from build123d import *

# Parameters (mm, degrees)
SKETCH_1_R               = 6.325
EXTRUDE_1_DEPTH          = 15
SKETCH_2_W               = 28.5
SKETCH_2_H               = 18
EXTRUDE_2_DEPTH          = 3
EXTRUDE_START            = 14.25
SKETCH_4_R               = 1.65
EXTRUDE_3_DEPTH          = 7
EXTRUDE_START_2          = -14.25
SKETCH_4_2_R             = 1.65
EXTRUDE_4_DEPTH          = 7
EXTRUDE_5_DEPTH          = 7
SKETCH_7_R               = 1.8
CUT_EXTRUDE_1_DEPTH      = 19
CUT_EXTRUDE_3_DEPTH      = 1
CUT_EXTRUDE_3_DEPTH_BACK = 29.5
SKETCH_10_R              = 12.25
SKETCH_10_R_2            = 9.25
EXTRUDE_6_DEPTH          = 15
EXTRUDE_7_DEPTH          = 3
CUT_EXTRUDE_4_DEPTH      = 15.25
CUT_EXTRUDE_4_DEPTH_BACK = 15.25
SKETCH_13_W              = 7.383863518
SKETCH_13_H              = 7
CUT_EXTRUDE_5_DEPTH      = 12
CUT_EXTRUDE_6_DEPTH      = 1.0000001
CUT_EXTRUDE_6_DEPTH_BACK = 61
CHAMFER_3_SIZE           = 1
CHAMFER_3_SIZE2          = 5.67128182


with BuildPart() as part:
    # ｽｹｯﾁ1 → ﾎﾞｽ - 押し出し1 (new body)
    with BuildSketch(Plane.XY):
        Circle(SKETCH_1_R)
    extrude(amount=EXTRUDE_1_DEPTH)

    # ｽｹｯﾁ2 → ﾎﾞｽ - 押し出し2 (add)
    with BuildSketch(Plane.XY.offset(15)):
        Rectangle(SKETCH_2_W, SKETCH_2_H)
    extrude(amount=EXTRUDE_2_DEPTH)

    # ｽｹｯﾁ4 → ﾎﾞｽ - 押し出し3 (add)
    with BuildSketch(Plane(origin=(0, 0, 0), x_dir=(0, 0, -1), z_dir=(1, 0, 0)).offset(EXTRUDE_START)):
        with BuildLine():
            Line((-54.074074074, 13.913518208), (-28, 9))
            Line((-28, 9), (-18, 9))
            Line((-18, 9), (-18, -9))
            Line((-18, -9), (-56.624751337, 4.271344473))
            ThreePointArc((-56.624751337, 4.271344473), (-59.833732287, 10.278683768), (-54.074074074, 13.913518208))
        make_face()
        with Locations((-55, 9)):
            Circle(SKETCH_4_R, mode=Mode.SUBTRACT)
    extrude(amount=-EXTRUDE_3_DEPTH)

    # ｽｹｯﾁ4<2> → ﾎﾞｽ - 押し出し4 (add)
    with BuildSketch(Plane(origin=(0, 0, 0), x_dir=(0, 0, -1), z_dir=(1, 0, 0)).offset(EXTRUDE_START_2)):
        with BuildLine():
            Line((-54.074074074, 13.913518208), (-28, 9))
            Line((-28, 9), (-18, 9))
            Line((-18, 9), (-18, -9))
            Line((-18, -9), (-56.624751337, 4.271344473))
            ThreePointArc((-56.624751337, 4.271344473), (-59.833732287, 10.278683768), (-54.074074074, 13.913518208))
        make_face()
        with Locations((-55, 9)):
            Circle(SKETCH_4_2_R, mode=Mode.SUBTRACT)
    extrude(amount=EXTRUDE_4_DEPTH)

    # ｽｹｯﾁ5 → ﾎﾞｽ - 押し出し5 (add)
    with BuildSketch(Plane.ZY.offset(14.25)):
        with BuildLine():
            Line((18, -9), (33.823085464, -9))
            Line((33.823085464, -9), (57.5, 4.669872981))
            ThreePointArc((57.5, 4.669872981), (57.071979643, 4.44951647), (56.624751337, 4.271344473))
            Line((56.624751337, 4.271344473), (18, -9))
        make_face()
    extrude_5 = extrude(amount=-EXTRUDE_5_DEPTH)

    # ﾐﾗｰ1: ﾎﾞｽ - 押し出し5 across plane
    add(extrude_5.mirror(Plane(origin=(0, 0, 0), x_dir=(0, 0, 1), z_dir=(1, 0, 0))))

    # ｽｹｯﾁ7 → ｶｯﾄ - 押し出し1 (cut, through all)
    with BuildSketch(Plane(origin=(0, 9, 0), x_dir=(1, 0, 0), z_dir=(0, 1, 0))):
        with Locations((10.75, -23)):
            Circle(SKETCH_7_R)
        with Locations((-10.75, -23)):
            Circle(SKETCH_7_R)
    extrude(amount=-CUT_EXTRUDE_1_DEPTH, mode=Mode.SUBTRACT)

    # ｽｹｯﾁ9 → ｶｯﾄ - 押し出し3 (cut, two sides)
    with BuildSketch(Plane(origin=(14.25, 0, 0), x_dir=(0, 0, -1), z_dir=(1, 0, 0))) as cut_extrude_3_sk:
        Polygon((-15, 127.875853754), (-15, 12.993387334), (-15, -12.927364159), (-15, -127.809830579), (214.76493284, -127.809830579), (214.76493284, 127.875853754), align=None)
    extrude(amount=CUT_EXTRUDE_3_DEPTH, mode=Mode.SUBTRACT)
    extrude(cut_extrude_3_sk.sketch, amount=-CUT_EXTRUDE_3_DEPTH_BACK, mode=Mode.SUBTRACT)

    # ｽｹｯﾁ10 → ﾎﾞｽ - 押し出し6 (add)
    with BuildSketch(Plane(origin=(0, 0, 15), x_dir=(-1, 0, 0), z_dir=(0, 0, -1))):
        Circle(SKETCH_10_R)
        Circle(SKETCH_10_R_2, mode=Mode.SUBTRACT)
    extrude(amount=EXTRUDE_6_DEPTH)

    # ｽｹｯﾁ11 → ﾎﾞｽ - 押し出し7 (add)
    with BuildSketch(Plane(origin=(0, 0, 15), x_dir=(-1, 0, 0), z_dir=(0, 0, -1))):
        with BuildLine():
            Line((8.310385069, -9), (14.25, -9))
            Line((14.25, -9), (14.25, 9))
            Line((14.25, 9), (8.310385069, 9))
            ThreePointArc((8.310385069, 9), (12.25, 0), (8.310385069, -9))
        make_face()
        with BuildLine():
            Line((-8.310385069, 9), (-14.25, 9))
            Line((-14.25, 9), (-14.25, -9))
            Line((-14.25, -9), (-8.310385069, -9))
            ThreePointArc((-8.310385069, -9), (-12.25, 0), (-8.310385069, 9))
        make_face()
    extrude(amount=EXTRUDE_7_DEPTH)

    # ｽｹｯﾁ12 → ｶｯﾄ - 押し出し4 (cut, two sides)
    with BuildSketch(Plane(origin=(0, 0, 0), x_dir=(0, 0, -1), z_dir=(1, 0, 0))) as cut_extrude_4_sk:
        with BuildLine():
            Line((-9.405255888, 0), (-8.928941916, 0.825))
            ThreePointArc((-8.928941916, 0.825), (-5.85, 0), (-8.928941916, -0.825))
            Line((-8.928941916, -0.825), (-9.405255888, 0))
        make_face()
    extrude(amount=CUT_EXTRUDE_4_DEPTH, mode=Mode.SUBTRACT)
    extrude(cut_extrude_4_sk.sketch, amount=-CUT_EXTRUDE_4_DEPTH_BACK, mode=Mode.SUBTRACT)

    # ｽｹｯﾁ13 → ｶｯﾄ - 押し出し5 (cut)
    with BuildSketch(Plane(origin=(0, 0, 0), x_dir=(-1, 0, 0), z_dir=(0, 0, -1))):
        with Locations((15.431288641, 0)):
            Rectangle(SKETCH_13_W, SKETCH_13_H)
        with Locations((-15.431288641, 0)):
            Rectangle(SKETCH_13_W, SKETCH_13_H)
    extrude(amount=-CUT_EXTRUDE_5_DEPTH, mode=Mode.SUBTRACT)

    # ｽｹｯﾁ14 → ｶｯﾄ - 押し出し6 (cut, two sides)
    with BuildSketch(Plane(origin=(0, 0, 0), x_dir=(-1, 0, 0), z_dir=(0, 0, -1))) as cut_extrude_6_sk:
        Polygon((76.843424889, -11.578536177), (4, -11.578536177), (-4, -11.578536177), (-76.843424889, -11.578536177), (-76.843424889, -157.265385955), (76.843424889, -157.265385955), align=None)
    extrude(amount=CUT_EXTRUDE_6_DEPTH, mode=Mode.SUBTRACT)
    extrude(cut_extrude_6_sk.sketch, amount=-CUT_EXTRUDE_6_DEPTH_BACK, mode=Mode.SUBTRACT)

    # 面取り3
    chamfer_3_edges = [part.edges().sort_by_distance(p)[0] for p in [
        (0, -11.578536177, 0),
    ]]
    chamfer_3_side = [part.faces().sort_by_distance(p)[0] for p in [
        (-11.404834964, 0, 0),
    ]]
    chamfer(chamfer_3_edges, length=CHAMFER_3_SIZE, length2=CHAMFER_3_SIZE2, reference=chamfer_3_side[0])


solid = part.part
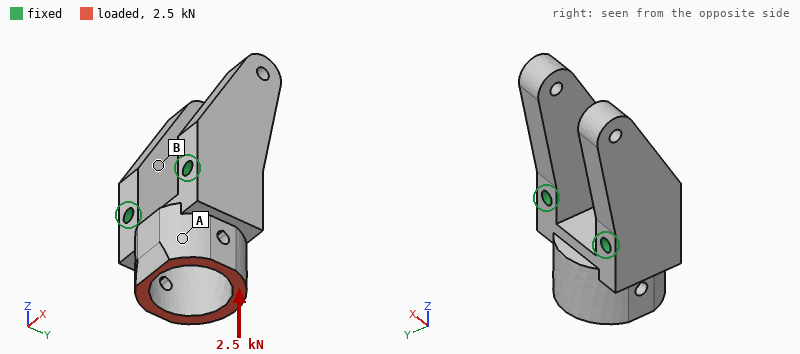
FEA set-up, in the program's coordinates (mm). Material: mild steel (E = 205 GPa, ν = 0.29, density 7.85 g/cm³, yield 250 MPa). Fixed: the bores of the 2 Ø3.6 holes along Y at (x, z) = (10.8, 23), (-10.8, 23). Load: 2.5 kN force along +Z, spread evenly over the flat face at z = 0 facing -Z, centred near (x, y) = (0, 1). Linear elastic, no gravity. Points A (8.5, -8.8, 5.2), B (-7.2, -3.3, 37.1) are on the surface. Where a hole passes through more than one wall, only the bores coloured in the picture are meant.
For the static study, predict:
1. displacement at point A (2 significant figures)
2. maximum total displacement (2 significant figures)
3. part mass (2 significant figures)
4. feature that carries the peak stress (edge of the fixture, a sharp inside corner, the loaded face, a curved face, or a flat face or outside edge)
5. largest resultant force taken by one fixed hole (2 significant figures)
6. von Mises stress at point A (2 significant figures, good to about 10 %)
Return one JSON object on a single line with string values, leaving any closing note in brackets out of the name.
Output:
{"displacement at point A": "1.3 µm", "maximum total displacement": "4.3 µm", "part mass": "100 g", "feature that carries the peak stress": "a curved face", "largest resultant force taken by one fixed hole": "1.3 kN", "von Mises stress at point A": "16 MPa"}
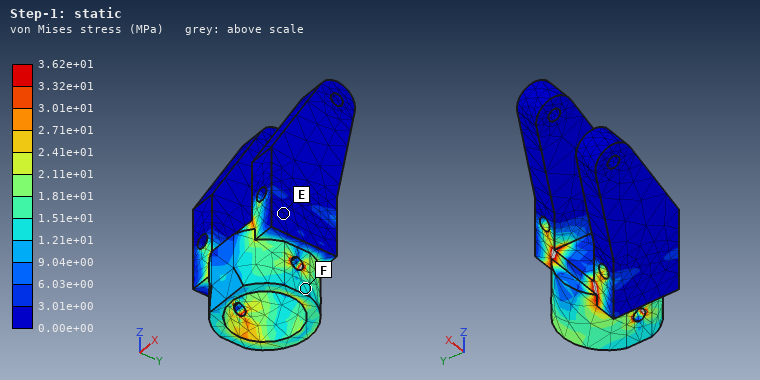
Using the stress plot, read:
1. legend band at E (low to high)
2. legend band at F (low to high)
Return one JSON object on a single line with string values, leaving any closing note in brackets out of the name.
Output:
{"legend band at E": "0.00e+00 to 3.01e+00 MPa", "legend band at F": "1.21e+01 to 1.51e+01 MPa"}
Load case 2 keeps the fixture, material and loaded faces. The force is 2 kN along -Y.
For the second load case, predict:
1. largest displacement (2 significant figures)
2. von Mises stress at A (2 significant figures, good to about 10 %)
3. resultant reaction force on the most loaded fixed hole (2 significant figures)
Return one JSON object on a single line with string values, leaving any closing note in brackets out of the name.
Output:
{"largest displacement": "18 µm", "von Mises stress at A": "26 MPa", "resultant reaction force on the most loaded fixed hole": "1.0 kN"}
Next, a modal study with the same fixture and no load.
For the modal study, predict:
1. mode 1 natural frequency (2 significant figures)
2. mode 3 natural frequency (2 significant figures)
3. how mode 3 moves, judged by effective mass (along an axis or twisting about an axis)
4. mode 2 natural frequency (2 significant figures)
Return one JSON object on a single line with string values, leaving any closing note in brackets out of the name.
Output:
{"mode 1 natural frequency": "5100 Hz", "mode 3 natural frequency": "12 kHz", "how mode 3 moves, judged by effective mass": "along Y", "mode 2 natural frequency": "5100 Hz"}
